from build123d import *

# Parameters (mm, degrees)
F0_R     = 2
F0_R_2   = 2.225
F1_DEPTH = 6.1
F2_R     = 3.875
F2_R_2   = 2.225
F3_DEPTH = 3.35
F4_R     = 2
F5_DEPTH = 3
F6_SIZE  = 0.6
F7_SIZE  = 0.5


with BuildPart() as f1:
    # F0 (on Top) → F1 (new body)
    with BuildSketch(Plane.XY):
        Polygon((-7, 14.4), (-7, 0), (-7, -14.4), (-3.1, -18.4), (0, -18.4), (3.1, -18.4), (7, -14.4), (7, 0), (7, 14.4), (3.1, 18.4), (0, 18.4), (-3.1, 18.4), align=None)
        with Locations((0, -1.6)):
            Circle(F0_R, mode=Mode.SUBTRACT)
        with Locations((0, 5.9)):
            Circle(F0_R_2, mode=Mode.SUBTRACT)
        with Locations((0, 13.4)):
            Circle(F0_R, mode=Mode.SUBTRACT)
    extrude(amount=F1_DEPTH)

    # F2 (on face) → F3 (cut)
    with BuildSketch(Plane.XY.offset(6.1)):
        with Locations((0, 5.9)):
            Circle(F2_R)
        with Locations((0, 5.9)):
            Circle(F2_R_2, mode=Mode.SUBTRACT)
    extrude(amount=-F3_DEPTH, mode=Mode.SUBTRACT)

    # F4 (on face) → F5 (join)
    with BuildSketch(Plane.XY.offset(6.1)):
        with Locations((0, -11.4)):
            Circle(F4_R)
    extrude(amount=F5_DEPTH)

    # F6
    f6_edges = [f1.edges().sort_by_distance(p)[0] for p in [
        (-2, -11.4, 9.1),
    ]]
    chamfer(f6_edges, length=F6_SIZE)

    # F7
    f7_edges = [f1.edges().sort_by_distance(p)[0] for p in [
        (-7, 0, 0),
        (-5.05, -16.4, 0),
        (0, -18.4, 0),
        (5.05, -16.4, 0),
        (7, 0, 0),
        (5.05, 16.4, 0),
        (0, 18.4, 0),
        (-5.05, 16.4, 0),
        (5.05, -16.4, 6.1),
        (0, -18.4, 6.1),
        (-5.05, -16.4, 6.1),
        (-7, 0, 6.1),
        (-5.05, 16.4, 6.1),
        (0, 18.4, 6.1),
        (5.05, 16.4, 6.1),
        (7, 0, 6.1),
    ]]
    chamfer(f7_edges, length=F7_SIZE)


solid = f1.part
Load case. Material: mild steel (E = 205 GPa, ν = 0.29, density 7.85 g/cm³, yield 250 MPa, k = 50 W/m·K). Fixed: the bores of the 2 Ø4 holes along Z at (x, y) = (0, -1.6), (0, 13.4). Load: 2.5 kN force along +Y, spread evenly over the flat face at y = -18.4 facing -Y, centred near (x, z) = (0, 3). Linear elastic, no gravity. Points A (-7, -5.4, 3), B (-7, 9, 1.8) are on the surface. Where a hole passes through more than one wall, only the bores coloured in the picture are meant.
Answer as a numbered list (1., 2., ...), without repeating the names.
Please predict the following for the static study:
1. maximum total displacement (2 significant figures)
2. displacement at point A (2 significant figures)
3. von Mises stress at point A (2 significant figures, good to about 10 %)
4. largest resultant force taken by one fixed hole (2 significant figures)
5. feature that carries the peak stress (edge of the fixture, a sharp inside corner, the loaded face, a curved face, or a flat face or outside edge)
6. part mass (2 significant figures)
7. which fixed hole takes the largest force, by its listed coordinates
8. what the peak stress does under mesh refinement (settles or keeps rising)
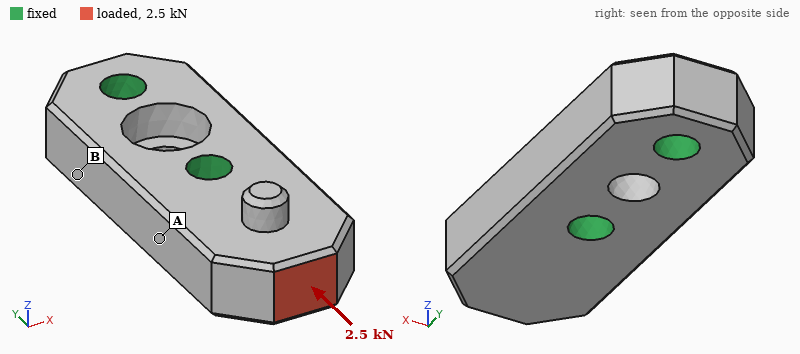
1. 3.7 µm
2. 0.99 µm
3. 16 MPa
4. 2.2 kN
5. edge of the fixture
6. 20 g
7. (0, -1.6)
8. keeps rising
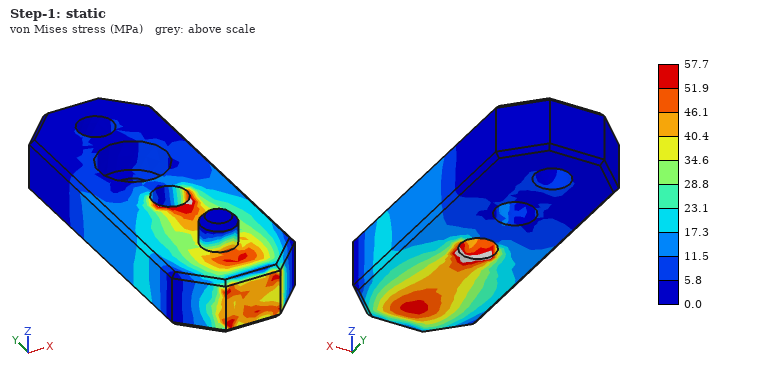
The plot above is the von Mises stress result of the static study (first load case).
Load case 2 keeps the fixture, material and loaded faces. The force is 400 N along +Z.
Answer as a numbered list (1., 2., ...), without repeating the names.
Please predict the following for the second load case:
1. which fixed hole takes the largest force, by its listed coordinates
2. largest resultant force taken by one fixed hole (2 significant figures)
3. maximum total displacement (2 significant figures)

1. (0, -1.6)
2. 470 N
3. 13 µm
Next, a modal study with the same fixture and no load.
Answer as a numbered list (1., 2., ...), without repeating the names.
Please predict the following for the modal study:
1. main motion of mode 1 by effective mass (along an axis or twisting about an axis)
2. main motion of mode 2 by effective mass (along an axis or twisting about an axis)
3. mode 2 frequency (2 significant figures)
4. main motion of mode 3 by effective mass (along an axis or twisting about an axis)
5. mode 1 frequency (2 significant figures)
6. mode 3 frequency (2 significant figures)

1. along Z
2. along X
3. 25 kHz
4. twisting about Y
5. 19 kHz
6. 38 kHz
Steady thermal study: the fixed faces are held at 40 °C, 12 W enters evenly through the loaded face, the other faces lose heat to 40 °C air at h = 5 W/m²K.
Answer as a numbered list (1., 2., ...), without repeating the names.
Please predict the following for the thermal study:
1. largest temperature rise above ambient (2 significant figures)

1. 58 K
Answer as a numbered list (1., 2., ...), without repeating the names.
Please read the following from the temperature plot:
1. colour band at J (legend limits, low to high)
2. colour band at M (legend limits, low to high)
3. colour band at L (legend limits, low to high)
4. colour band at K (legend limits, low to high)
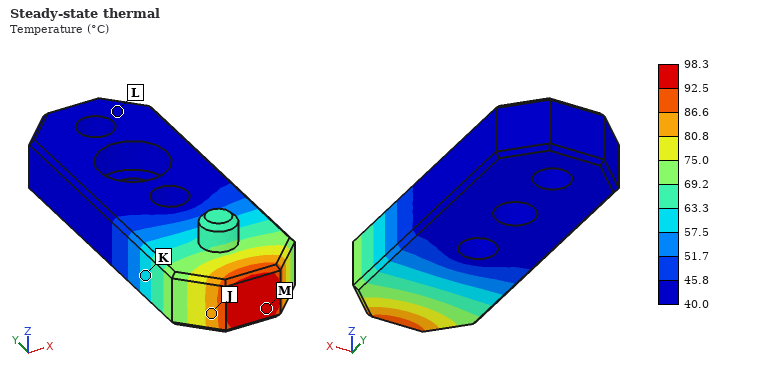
1. 80.8 to 86.6 °C
2. 92.5 to 98.3 °C
3. 40.0 to 45.8 °C
4. 57.5 to 63.3 °C
